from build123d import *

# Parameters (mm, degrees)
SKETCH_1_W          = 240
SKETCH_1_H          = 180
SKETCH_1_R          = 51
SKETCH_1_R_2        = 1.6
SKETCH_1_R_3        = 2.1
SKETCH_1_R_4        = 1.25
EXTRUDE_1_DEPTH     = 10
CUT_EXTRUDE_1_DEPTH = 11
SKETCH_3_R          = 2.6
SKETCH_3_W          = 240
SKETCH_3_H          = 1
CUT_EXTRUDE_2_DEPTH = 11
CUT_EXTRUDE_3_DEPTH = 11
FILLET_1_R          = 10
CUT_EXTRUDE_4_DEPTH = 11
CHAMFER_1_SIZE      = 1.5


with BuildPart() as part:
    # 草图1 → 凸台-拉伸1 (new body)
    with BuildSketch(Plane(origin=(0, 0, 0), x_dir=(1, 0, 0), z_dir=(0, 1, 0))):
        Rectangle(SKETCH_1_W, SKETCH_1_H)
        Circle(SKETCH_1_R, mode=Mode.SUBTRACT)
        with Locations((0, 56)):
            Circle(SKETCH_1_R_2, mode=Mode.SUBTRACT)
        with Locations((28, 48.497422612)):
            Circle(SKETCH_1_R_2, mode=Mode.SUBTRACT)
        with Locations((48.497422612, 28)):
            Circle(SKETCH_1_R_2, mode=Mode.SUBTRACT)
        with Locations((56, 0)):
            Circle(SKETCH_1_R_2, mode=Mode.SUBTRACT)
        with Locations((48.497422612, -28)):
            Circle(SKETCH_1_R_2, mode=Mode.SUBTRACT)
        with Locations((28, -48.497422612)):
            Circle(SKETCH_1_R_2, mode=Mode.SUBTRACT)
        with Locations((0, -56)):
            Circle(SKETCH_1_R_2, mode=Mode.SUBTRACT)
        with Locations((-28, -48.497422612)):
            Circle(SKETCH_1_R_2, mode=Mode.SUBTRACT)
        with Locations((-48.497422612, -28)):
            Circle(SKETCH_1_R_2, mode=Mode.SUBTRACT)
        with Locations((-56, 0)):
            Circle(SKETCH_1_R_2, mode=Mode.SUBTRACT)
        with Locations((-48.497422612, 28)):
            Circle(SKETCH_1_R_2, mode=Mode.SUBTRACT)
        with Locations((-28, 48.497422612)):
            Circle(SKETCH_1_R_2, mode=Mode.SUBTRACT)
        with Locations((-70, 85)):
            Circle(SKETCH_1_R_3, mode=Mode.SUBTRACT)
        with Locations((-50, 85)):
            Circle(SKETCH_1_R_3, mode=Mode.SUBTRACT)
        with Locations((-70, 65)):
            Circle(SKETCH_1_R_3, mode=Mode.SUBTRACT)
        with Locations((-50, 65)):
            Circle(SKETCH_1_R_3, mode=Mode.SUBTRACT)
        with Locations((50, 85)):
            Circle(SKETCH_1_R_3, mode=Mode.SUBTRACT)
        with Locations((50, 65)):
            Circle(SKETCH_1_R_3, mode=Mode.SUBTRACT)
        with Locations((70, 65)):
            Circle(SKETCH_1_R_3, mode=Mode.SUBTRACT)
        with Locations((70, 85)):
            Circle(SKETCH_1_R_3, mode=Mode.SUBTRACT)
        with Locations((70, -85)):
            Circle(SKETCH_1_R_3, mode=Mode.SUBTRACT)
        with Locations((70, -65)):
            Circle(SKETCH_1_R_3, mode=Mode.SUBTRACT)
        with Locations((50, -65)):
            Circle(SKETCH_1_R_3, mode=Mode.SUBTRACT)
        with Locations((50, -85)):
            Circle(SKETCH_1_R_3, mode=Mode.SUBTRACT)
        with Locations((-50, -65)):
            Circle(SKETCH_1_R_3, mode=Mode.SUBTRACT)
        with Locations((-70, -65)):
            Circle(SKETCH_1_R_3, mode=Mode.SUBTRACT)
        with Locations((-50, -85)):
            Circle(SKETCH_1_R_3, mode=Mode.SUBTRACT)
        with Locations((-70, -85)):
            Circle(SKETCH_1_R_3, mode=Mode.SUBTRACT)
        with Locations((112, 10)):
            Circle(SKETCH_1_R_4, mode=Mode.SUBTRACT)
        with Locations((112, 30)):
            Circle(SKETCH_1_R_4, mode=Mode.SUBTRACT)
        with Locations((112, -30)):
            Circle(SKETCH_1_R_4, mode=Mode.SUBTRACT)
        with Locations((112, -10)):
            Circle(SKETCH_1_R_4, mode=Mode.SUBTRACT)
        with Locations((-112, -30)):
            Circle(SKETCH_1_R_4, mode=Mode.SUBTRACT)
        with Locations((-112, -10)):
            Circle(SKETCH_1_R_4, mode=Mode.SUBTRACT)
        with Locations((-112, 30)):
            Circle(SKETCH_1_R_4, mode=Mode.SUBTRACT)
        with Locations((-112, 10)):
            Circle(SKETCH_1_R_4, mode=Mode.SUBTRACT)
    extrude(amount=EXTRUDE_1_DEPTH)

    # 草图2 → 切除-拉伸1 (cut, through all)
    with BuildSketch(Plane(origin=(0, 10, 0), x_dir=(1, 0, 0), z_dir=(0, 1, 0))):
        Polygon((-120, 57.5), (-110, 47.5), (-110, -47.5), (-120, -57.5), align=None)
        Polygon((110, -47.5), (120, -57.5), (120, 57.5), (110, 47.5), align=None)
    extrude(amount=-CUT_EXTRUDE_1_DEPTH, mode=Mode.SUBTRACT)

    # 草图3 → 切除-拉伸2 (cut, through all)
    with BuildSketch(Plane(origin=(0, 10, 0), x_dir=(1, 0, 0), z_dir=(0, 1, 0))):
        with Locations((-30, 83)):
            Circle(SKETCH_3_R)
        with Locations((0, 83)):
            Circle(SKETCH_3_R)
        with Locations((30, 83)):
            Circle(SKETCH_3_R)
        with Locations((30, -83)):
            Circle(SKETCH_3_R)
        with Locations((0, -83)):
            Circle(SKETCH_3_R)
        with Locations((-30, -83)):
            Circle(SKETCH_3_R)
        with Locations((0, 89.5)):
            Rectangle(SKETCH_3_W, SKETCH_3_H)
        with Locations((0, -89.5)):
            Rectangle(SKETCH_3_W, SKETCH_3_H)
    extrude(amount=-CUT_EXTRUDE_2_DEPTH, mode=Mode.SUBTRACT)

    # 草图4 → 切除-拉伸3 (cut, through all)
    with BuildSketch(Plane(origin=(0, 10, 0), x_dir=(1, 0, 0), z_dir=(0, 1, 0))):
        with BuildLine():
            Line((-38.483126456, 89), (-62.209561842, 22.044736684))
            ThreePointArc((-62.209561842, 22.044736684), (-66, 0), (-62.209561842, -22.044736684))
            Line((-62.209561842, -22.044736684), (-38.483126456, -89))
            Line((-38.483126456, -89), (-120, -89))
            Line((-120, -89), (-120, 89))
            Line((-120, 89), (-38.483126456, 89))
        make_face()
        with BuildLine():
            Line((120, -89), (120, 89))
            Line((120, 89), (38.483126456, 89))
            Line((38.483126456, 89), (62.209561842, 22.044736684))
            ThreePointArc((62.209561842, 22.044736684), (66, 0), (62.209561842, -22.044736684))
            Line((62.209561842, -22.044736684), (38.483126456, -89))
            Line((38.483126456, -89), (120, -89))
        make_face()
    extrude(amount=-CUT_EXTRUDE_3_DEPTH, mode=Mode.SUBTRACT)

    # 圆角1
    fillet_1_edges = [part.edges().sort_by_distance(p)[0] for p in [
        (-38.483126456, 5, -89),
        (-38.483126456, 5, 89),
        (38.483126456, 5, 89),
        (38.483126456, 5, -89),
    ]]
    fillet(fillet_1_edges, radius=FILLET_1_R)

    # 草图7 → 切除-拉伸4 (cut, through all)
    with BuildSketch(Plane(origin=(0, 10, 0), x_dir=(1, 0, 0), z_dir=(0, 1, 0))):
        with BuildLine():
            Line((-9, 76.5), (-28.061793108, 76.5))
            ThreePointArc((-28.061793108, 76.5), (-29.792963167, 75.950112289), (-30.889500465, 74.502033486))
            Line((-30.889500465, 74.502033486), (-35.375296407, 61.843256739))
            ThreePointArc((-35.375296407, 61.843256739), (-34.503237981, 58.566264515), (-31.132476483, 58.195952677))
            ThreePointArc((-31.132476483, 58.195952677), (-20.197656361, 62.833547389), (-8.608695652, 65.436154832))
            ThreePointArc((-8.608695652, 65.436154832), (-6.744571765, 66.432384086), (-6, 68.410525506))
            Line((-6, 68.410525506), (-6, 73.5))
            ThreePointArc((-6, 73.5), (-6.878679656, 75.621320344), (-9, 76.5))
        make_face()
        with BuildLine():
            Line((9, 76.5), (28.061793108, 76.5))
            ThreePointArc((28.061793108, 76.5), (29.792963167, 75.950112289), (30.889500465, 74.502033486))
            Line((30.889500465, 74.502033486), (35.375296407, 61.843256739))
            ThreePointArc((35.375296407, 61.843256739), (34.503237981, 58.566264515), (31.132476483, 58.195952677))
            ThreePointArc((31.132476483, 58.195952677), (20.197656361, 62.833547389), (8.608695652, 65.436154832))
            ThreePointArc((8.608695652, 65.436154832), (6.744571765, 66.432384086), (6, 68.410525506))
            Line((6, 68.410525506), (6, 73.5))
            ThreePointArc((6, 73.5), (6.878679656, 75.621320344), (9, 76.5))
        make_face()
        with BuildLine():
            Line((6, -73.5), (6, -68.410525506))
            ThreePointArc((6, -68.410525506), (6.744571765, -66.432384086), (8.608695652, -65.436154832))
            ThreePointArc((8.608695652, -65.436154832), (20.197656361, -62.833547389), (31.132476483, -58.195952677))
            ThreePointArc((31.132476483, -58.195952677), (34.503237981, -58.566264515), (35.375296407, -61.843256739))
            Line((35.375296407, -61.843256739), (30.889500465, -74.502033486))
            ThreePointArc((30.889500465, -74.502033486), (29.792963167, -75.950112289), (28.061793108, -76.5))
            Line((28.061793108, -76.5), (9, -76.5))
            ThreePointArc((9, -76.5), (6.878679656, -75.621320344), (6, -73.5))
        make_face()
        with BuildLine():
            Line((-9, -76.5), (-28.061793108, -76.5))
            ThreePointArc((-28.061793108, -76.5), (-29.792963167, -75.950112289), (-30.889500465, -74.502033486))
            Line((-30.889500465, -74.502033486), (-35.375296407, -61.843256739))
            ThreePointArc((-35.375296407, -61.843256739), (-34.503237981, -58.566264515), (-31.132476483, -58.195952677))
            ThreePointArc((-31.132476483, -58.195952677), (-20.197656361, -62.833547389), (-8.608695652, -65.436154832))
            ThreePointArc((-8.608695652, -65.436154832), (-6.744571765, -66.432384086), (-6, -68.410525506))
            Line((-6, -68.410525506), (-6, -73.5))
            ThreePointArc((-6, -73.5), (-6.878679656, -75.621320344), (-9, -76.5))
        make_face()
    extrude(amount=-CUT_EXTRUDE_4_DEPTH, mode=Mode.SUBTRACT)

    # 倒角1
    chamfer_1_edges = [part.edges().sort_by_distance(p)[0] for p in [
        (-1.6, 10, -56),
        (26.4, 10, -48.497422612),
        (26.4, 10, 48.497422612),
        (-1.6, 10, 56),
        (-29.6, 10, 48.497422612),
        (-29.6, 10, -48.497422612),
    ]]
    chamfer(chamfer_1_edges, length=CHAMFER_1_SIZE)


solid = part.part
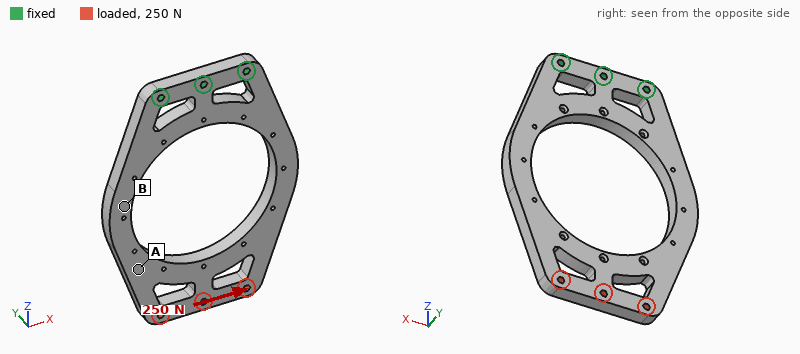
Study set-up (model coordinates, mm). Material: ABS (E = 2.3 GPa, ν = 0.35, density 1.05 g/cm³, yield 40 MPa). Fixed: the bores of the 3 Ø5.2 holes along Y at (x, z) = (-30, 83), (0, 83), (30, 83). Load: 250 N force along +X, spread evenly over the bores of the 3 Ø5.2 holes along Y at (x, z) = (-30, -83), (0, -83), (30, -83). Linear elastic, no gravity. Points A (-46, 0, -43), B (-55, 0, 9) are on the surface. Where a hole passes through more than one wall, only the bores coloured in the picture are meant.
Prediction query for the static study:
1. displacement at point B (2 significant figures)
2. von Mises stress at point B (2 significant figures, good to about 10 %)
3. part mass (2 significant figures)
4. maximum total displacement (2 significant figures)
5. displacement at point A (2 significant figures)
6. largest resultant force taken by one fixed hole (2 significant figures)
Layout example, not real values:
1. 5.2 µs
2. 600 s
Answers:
1. 1.1 mm
2. 3.0 MPa
3. 97 g
4. 2.4 mm
5. 2.1 mm
6. 600 N
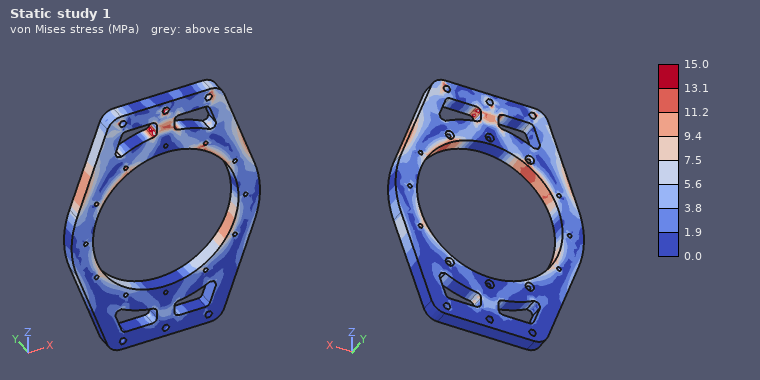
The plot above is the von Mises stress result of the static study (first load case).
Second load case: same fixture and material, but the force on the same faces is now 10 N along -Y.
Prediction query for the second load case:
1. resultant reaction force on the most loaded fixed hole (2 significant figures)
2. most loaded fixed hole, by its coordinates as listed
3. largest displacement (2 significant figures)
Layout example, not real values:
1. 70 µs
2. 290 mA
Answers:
1. 13 N
2. (0, 83)
3. 2.6 mm
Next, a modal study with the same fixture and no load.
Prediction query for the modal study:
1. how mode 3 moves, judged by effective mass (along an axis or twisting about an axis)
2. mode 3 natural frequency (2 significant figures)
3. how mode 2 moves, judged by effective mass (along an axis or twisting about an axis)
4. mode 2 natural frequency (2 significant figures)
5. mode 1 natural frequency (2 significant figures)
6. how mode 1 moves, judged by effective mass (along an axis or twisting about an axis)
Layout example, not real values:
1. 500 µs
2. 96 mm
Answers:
1. along X
2. 250 Hz
3. twisting about Z
4. 190 Hz
5. 60 Hz
6. along Y
